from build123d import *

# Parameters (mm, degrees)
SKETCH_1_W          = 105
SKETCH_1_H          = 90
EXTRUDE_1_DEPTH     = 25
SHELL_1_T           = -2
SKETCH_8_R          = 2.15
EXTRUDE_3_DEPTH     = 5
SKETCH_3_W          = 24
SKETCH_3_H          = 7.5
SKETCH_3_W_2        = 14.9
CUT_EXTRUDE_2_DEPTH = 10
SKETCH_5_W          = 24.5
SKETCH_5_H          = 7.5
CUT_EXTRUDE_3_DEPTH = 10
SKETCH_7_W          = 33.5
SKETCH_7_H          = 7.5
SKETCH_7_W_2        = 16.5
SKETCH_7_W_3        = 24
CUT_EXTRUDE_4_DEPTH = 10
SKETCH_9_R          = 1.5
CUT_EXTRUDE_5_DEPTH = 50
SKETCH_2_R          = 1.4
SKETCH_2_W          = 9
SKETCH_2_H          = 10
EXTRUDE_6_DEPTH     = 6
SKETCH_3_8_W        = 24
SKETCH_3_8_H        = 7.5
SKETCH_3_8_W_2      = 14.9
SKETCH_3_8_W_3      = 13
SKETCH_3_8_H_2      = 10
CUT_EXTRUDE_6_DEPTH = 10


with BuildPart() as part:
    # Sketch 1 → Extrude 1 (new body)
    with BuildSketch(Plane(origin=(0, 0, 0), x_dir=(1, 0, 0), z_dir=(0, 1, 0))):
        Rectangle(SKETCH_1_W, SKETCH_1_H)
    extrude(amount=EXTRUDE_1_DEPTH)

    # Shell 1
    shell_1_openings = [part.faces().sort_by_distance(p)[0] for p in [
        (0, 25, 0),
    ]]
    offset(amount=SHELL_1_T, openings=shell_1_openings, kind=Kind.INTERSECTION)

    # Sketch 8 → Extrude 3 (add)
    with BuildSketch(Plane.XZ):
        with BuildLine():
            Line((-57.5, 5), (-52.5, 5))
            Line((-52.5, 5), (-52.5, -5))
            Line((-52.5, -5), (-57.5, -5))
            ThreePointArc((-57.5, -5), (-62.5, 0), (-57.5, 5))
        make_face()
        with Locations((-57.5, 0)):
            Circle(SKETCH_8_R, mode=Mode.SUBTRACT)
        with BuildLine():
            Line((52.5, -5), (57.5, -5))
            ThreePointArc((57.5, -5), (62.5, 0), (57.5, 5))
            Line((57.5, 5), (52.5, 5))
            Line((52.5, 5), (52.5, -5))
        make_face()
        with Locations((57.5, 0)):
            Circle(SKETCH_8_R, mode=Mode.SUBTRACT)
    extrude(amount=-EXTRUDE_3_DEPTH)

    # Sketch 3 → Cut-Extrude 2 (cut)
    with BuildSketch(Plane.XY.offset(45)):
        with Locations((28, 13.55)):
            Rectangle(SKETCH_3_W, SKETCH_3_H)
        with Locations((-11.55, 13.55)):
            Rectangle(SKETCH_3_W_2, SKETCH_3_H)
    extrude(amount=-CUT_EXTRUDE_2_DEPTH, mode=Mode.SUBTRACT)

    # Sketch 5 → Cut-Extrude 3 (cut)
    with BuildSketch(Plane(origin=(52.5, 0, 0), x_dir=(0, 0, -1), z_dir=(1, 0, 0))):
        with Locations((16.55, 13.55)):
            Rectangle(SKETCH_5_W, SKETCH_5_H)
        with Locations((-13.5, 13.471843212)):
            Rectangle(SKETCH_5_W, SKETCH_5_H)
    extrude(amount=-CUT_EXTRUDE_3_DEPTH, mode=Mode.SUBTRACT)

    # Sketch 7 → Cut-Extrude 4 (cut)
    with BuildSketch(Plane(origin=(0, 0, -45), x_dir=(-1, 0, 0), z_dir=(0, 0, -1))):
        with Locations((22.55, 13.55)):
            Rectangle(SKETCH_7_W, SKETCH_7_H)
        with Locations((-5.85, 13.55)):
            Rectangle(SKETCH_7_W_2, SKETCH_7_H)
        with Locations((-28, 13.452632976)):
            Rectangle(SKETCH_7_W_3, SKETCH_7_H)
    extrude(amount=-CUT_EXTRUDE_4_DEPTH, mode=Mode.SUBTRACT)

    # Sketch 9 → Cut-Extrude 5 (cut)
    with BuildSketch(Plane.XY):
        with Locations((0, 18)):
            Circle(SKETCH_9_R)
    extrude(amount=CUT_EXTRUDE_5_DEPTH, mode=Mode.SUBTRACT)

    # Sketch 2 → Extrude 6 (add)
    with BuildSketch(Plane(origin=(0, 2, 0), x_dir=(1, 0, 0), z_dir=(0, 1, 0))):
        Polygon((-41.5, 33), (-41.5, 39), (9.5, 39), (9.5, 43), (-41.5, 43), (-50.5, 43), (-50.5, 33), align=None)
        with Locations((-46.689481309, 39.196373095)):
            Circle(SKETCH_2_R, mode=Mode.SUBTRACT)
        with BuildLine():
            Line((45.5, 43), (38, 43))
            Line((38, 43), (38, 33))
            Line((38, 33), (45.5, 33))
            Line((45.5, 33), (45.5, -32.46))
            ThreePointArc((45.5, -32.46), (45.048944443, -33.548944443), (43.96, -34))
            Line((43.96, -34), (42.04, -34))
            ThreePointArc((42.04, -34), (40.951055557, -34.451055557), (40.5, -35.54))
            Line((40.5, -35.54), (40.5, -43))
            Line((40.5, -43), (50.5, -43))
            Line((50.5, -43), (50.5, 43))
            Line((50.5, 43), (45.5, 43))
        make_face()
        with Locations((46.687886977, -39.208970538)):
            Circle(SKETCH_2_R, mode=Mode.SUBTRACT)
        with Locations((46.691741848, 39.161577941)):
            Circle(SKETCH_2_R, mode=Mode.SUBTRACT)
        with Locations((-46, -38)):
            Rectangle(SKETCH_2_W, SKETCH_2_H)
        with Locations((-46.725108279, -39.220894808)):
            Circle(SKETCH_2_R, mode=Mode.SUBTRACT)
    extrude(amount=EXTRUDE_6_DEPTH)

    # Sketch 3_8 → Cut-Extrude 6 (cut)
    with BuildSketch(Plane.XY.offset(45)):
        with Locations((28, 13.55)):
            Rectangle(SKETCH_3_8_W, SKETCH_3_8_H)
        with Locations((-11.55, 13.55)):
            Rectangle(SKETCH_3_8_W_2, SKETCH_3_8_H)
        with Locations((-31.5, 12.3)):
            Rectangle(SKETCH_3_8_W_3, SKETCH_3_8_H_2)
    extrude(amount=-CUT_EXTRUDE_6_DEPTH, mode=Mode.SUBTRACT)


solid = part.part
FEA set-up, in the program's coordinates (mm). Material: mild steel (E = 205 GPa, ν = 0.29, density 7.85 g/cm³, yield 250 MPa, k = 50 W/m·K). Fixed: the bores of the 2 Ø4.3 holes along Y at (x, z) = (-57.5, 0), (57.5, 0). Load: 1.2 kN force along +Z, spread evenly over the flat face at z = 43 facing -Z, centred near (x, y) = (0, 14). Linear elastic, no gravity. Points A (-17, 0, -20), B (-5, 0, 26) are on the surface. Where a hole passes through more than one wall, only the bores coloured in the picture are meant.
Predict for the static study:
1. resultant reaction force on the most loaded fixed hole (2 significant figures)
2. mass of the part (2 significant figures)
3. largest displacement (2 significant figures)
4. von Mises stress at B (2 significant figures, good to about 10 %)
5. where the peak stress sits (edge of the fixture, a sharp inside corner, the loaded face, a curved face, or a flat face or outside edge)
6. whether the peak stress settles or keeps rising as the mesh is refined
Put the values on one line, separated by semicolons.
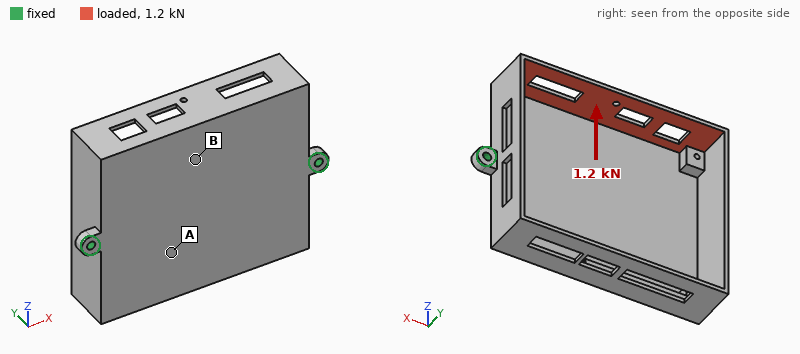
610 N; 310 g; 0.38 mm; 46 MPa; edge of the fixture; keeps rising
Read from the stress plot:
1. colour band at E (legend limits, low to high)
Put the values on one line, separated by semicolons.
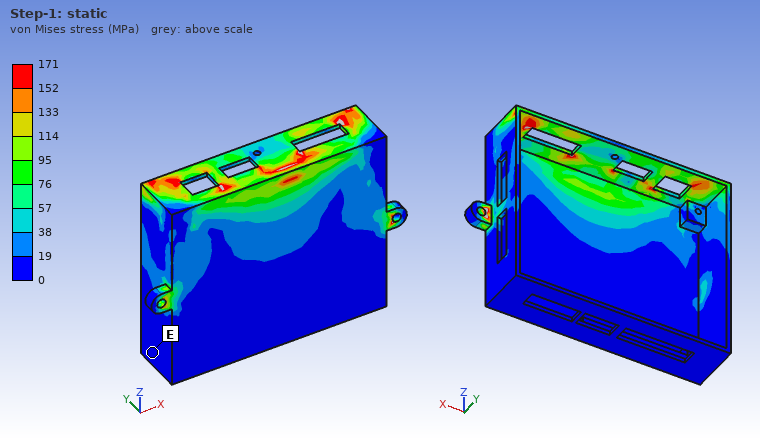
0 to 19 MPa
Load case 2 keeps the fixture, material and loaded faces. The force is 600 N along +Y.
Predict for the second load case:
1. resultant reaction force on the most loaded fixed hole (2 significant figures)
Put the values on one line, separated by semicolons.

320 N
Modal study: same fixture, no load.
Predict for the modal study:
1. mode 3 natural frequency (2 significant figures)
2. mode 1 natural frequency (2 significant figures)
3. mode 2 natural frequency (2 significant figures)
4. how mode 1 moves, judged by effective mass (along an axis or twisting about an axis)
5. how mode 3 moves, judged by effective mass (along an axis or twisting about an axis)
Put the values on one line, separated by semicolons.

1600 Hz; 820 Hz; 1300 Hz; twisting about X; along Y
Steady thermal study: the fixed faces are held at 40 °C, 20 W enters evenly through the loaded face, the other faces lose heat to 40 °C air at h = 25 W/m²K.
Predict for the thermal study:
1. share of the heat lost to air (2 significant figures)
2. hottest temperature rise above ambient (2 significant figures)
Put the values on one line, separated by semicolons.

73 %; 76 K
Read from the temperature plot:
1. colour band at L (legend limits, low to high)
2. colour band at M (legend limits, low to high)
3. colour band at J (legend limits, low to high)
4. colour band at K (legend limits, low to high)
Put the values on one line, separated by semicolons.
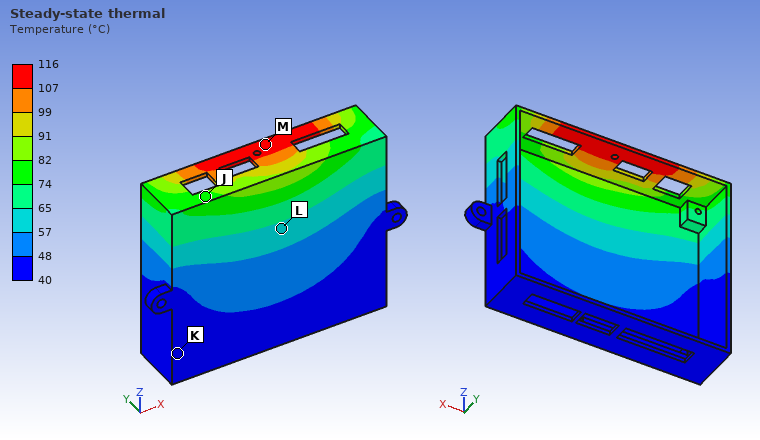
57 to 65 °C; 107 to 116 °C; 74 to 82 °C; 40 to 48 °C
